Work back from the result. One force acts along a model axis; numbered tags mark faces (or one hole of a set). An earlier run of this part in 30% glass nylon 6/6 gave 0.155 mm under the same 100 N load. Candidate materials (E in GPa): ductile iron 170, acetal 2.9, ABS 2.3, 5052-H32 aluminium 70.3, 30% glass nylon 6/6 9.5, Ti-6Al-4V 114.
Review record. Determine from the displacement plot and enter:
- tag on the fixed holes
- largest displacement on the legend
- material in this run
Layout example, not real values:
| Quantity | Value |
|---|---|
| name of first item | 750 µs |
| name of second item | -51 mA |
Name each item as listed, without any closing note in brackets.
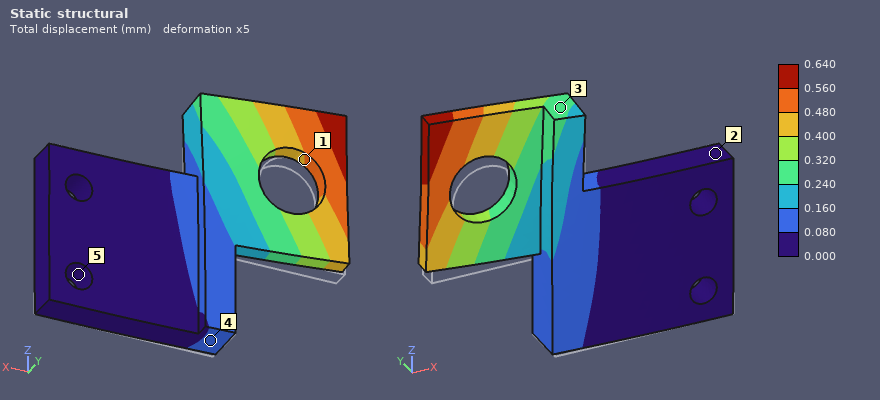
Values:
| Quantity | Value |
|---|---|
| tag on the fixed holes | 5 |
| largest displacement on the legend | 0.640 mm |
| material in this run | ABS |
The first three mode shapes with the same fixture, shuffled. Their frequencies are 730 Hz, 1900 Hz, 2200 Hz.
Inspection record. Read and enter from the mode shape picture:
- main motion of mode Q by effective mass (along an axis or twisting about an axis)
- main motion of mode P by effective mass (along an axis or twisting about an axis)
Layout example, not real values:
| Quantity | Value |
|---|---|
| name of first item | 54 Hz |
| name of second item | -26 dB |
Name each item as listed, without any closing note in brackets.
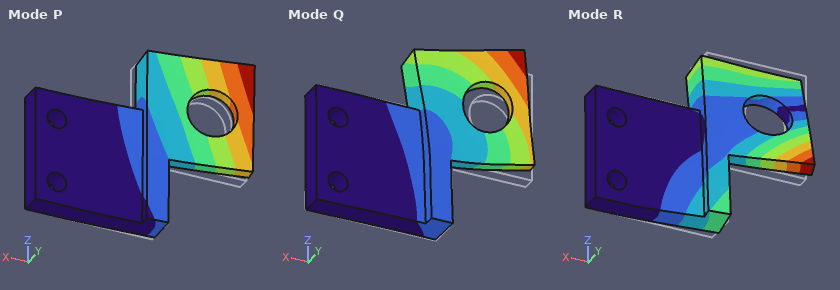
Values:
| Quantity | Value |
|---|---|
| main motion of mode Q by effective mass | along Z |
| main motion of mode P by effective mass | along Y |
